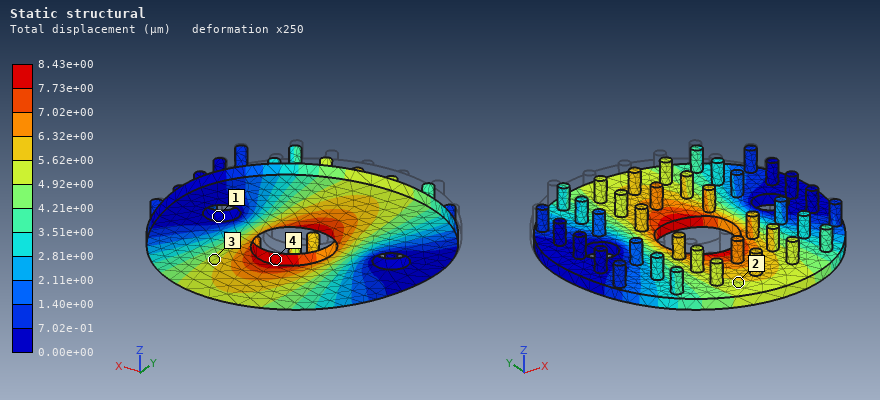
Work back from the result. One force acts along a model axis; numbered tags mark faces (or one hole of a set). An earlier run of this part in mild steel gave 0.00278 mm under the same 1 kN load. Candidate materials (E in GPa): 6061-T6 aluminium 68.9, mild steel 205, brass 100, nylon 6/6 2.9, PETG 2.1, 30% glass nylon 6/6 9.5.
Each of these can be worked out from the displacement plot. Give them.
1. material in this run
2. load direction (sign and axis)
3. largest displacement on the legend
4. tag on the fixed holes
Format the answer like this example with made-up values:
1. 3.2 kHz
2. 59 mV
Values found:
1. 6061-T6 aluminium
2. -Y
3. 8.43e+00 µm
4. 1
